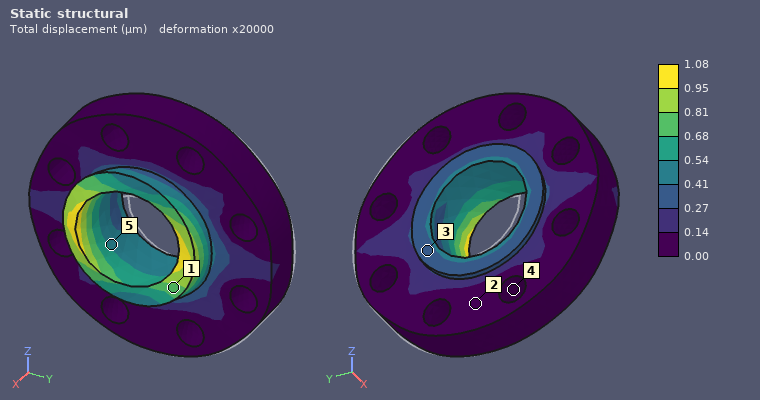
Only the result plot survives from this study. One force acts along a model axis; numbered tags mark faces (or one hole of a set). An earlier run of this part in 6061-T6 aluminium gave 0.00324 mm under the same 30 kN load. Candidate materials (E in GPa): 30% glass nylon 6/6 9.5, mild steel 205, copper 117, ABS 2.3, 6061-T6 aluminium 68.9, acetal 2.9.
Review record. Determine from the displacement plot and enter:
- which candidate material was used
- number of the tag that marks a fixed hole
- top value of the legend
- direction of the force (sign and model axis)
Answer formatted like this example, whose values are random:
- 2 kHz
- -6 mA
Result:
- mild steel
- 4
- 1.08 µm
- -Y
